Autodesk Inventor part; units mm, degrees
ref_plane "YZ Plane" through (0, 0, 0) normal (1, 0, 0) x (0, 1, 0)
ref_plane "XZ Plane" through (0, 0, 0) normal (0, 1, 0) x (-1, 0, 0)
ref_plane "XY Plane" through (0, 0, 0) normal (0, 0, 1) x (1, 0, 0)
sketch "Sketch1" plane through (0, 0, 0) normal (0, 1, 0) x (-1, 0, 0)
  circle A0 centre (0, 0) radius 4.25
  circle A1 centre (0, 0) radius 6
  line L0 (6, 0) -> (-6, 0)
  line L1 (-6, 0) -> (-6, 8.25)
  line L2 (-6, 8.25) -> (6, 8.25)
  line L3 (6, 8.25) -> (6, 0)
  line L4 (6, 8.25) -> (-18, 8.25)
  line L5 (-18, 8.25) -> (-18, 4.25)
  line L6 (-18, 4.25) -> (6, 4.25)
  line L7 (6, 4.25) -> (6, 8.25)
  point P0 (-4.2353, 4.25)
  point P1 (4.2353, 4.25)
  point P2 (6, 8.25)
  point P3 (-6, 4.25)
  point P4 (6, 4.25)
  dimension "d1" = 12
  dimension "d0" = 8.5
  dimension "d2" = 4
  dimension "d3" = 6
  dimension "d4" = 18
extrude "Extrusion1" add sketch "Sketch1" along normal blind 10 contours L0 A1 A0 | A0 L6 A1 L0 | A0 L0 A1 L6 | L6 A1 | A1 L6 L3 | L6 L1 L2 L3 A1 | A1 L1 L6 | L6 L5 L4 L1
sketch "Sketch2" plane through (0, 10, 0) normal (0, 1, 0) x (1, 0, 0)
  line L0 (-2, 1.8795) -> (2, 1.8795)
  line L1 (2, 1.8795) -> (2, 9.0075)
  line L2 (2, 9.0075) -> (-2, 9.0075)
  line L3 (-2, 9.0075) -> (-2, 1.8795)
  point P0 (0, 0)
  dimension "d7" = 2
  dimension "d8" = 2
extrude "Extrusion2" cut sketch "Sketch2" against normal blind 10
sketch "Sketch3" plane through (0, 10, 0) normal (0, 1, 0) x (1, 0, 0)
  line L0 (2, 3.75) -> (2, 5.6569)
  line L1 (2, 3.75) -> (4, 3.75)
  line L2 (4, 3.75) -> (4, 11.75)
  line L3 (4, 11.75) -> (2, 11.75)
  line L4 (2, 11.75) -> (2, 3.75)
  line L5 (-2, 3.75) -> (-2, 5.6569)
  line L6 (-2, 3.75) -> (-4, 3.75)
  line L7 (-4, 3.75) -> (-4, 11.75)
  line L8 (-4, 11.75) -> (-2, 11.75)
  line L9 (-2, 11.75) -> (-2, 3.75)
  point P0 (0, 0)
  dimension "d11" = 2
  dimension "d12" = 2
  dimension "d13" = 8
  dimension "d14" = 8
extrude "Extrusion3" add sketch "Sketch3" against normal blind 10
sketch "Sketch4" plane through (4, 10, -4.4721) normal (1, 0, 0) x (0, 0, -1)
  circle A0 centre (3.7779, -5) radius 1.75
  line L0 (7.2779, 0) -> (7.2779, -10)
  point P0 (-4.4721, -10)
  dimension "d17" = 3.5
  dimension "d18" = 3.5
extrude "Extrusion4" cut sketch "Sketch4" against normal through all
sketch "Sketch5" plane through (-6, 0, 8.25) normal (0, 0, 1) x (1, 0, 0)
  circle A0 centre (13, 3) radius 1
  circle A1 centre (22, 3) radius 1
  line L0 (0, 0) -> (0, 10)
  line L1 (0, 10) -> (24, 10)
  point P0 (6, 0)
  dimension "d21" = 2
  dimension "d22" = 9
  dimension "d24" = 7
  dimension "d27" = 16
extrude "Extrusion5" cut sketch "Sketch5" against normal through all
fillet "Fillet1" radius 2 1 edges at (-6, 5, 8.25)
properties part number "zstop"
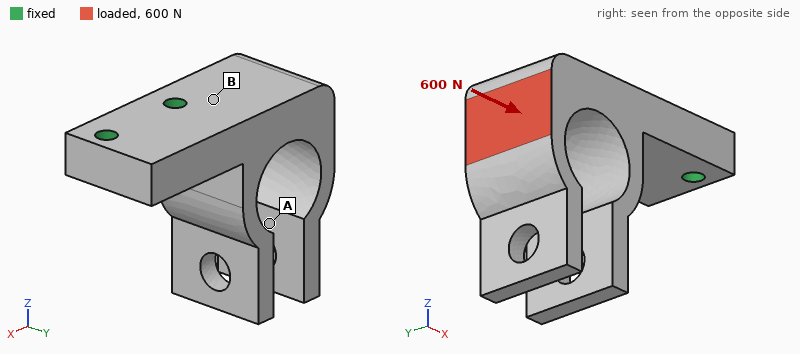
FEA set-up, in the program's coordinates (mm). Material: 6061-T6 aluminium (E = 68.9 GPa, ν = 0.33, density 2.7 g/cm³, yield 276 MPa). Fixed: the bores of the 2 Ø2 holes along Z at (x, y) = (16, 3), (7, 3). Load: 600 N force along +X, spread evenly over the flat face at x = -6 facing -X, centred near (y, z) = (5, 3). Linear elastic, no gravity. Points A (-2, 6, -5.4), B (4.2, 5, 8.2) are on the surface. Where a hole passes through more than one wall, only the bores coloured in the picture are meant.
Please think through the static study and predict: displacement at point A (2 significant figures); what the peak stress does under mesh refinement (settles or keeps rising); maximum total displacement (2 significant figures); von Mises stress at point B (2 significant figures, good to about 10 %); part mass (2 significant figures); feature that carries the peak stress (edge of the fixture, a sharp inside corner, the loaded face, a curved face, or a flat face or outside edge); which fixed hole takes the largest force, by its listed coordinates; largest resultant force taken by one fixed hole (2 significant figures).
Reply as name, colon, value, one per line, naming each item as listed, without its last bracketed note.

displacement at point A: 0.066 mm
what the peak stress does under mesh refinement: keeps rising
maximum total displacement: 0.10 mm
von Mises stress at point B: 35 MPa
part mass: 4.3 g
feature that carries the peak stress: edge of the fixture
which fixed hole takes the largest force, by its listed coordinates: (7, 3)
largest resultant force taken by one fixed hole: 500 N
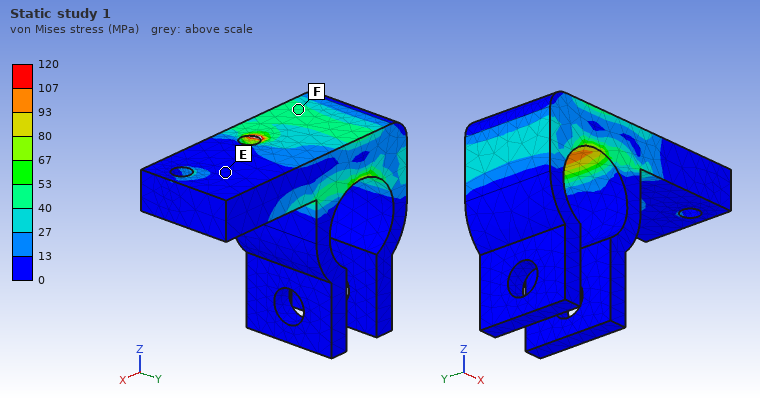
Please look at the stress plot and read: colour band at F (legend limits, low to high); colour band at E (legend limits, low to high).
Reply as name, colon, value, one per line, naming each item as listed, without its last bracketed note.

colour band at F: 40 to 53 MPa
colour band at E: 0 to 13 MPa
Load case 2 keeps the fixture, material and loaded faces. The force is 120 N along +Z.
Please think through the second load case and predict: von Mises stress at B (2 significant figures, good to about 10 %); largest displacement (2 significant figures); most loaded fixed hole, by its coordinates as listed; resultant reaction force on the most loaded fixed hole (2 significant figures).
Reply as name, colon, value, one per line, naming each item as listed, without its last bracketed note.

von Mises stress at B: 36 MPa
largest displacement: 51 µm
most loaded fixed hole, by its coordinates as listed: (7, 3)
resultant reaction force on the most loaded fixed hole: 170 N
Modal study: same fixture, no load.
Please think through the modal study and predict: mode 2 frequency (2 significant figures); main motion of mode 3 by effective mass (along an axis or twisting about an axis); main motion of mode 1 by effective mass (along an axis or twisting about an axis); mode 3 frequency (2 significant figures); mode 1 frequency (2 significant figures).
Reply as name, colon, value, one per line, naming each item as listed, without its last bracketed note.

mode 2 frequency: 6500 Hz
main motion of mode 3 by effective mass: along Y
main motion of mode 1 by effective mass: along X
mode 3 frequency: 8700 Hz
mode 1 frequency: 5600 Hz
